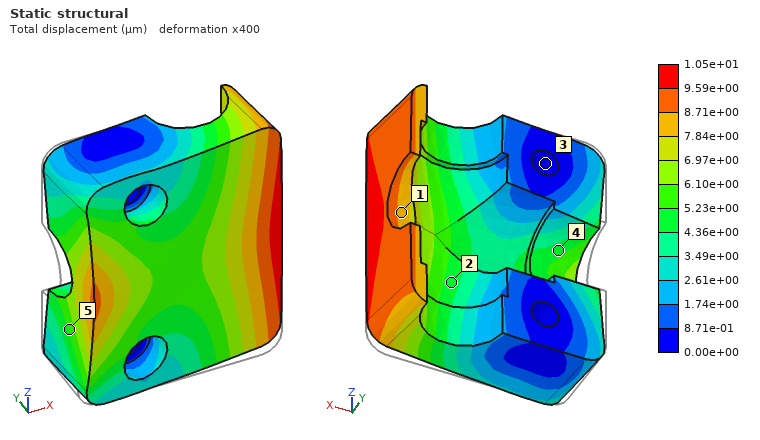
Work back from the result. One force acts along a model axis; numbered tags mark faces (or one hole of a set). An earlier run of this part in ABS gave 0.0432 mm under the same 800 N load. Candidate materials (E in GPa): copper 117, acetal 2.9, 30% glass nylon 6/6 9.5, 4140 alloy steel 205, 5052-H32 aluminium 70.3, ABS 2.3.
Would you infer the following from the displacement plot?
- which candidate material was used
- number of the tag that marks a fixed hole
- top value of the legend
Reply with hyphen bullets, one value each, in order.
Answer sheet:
- 30% glass nylon 6/6
- 3
- 1.05e+01 µm
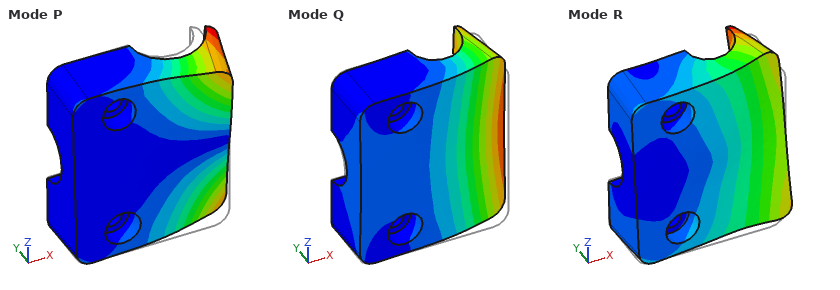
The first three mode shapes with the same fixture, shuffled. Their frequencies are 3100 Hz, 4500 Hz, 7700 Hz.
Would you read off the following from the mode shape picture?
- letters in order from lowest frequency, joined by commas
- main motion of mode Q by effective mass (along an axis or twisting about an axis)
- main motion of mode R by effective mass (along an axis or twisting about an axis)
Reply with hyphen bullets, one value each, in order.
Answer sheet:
- Q, P, R
- along Y
- along Z
